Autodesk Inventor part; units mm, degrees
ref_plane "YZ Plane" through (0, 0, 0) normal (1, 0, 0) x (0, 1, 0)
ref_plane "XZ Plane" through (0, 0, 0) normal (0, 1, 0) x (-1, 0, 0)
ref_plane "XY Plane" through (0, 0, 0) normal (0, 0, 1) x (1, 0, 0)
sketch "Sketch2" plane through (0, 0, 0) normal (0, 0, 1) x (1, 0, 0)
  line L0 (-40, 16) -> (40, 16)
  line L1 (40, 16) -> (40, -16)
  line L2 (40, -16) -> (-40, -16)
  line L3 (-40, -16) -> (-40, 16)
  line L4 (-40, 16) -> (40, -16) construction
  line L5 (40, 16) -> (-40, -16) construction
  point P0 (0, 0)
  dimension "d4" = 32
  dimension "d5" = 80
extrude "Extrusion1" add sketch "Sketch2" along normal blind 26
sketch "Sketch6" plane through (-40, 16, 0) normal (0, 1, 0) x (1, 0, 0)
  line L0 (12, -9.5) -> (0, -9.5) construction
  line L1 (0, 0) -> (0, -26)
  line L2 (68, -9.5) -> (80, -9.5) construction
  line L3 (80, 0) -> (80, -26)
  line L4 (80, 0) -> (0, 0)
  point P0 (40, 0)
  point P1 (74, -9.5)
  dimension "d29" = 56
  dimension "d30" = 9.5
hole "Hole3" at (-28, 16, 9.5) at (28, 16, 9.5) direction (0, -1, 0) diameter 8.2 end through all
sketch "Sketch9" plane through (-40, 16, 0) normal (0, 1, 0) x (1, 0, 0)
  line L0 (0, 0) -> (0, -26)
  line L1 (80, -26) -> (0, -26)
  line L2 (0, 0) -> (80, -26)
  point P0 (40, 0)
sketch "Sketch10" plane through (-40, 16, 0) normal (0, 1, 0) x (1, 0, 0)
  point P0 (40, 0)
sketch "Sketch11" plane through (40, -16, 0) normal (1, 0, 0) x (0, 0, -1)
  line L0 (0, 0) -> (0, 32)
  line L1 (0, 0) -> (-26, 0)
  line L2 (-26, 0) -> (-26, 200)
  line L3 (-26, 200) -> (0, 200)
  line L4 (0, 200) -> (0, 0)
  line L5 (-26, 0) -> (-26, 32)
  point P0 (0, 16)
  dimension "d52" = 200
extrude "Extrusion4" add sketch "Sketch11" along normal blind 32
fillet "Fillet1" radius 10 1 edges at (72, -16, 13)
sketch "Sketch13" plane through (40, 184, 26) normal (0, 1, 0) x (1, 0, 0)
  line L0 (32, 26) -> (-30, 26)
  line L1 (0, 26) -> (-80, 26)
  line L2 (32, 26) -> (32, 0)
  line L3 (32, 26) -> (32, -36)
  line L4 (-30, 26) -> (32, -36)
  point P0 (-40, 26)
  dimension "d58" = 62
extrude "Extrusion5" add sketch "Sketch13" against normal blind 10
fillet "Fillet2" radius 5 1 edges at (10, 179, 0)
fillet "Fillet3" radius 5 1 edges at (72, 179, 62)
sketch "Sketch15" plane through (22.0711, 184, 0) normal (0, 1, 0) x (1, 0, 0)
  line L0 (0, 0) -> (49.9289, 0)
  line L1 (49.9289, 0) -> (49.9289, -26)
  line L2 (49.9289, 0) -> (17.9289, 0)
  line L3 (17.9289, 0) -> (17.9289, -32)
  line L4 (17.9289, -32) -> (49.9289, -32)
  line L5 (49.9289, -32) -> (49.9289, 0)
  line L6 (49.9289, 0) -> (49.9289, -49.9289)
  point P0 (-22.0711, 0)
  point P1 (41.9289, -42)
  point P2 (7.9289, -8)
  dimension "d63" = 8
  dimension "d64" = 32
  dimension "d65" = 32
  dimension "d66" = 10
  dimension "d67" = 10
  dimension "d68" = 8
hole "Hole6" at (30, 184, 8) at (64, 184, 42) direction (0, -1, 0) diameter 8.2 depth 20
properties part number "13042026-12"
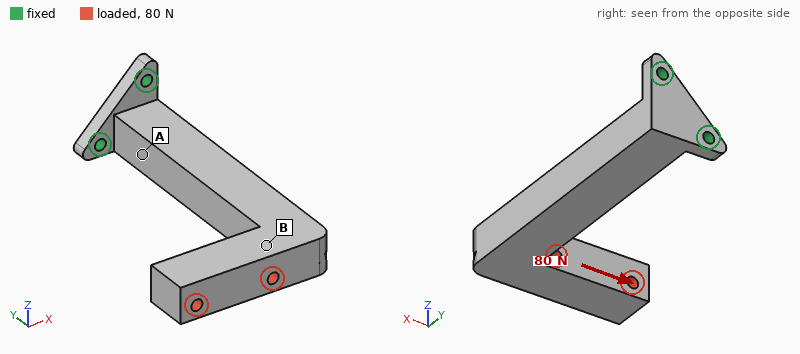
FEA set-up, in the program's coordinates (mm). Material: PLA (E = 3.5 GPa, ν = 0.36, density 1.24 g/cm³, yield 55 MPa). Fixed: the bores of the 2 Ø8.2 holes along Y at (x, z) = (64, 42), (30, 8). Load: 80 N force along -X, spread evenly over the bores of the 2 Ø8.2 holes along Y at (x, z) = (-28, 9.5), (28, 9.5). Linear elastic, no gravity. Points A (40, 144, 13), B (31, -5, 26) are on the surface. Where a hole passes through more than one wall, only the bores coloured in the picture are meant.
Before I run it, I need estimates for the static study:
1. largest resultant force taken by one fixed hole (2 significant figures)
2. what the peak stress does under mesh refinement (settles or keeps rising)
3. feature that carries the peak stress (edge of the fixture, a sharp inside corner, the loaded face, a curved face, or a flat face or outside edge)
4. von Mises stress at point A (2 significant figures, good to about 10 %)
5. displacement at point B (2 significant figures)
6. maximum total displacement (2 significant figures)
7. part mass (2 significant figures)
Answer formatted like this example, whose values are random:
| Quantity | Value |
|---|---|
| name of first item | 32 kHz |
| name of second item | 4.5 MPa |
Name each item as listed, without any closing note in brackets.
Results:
| Quantity | Value |
|---|---|
| largest resultant force taken by one fixed hole | 280 N |
| what the peak stress does under mesh refinement | keeps rising |
| feature that carries the peak stress | edge of the fixture |
| von Mises stress at point A | 2.6 MPa |
| displacement at point B | 2.1 mm |
| maximum total displacement | 2.5 mm |
| part mass | 300 g |
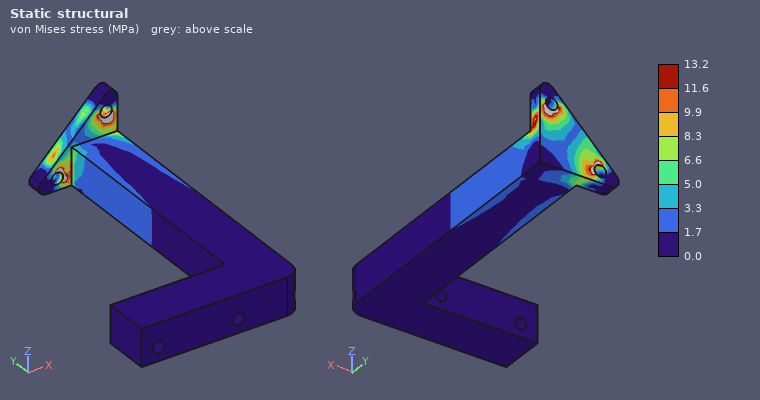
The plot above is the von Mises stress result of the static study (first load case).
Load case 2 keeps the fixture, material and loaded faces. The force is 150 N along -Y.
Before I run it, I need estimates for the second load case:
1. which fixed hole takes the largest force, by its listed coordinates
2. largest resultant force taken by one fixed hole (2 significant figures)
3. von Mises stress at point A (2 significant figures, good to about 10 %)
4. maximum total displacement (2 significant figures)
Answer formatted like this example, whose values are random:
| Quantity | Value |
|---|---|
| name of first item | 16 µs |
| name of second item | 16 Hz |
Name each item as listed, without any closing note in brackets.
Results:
| Quantity | Value |
|---|---|
| which fixed hole takes the largest force, by its listed coordinates | (30, 8) |
| largest resultant force taken by one fixed hole | 250 N |
| von Mises stress at point A | 2.1 MPa |
| maximum total displacement | 1.5 mm |
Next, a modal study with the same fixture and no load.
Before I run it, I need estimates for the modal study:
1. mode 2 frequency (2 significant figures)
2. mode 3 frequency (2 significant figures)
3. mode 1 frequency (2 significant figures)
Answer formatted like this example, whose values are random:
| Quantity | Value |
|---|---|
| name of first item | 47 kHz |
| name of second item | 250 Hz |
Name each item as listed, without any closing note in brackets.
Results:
| Quantity | Value |
|---|---|
| mode 2 frequency | 100 Hz |
| mode 3 frequency | 320 Hz |
| mode 1 frequency | 66 Hz |
